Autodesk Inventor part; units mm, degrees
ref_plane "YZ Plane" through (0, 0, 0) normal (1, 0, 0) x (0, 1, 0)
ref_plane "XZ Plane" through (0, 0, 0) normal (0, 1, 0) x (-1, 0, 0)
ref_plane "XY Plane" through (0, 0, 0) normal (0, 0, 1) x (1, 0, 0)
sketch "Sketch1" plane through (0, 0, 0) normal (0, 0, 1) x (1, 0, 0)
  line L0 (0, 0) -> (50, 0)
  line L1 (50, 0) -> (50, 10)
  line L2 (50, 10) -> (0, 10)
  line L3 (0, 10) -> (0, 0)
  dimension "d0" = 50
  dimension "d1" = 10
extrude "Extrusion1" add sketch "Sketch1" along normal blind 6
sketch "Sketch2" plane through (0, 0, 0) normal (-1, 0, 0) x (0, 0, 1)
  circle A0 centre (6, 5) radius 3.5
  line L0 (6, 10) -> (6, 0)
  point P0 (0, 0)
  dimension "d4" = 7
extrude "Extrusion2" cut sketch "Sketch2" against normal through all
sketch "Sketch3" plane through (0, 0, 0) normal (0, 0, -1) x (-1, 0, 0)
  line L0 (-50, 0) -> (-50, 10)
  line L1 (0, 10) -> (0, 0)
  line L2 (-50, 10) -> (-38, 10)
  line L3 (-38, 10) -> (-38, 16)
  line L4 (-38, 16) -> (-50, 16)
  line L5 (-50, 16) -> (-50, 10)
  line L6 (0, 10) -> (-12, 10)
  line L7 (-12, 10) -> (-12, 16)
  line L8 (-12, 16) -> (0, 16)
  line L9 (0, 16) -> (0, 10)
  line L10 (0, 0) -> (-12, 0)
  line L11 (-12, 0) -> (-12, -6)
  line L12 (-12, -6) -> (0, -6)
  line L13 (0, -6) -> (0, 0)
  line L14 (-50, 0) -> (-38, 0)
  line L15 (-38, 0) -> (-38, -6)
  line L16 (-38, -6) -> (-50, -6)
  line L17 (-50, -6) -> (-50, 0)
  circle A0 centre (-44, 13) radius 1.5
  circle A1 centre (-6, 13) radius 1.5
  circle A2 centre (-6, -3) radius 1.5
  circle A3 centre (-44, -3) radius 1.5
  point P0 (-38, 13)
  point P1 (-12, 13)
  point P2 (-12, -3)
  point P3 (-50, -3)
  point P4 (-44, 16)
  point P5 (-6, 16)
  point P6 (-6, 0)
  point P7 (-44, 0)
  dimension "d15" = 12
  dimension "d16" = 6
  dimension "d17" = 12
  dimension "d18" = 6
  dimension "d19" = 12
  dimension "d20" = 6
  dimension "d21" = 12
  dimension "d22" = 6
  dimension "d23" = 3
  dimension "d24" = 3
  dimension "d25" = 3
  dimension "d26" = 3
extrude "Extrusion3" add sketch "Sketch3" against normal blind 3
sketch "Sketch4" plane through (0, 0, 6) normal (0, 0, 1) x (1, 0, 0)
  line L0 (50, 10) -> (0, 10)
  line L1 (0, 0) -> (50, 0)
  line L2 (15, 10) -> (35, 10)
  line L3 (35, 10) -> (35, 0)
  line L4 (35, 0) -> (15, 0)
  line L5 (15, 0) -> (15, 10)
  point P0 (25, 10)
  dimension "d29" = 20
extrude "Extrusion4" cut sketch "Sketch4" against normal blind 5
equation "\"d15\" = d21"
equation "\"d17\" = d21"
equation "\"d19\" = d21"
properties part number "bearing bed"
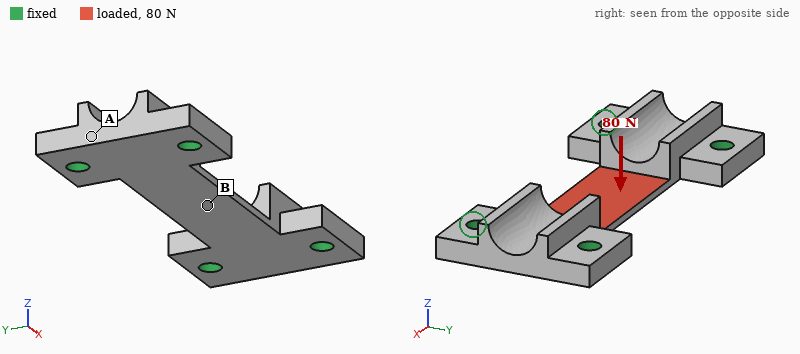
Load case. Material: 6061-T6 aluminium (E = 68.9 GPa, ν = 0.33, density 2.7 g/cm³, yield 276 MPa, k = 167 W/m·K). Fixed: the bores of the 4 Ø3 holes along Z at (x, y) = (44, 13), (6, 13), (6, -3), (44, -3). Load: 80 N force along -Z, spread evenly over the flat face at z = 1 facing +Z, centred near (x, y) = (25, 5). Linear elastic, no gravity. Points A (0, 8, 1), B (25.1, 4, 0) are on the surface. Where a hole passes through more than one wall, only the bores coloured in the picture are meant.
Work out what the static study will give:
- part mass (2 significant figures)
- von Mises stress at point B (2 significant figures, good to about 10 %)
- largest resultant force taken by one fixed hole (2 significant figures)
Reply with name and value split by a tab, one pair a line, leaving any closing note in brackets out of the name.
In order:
part mass	5.9 g
von Mises stress at point B	46 MPa
largest resultant force taken by one fixed hole	30 N
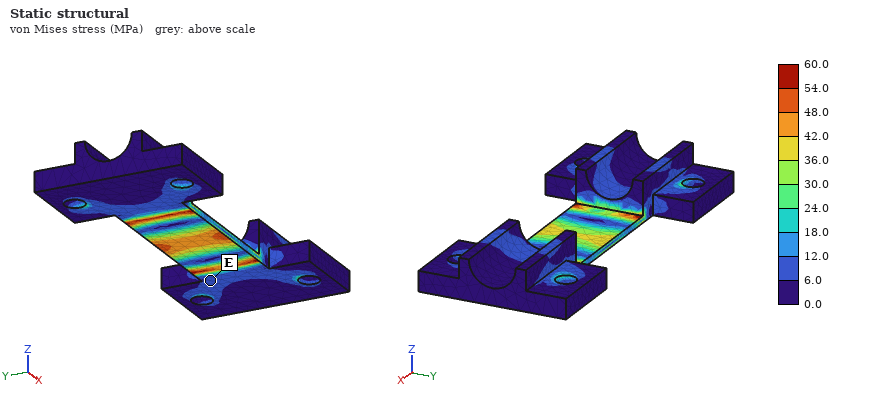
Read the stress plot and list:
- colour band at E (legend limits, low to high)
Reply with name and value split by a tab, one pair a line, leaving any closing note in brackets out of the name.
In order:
colour band at E	6.0 to 12.0 MPa
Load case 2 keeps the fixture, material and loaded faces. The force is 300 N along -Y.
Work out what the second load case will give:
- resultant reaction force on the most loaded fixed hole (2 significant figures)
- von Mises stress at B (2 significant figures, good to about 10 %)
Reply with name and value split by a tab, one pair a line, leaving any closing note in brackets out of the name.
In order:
resultant reaction force on the most loaded fixed hole	120 N
von Mises stress at B	6.8 MPa
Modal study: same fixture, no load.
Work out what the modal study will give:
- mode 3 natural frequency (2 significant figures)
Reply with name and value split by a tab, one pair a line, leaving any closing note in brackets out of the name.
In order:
mode 3 natural frequency	22 kHz
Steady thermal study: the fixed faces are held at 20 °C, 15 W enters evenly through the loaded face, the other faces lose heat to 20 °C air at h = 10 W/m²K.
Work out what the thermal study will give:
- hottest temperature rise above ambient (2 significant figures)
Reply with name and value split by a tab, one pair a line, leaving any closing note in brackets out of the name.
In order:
hottest temperature rise above ambient	35 K
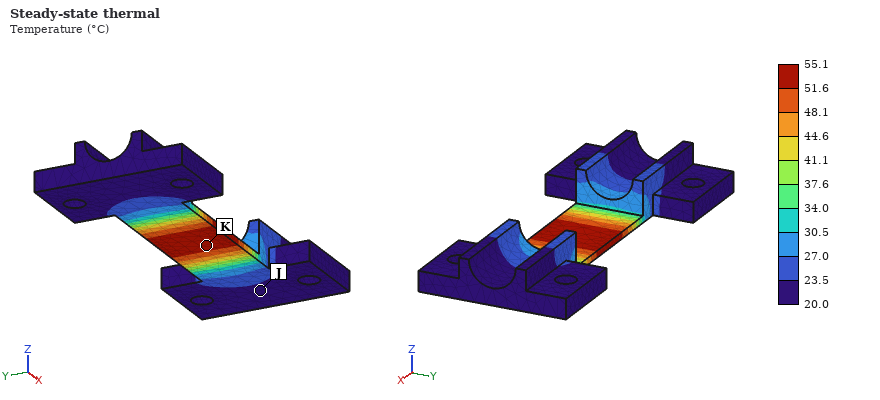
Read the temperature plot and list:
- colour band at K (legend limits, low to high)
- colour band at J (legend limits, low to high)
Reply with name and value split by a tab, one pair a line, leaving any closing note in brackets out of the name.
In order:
colour band at K	51.6 to 55.1 °C
colour band at J	20.0 to 23.5 °C
